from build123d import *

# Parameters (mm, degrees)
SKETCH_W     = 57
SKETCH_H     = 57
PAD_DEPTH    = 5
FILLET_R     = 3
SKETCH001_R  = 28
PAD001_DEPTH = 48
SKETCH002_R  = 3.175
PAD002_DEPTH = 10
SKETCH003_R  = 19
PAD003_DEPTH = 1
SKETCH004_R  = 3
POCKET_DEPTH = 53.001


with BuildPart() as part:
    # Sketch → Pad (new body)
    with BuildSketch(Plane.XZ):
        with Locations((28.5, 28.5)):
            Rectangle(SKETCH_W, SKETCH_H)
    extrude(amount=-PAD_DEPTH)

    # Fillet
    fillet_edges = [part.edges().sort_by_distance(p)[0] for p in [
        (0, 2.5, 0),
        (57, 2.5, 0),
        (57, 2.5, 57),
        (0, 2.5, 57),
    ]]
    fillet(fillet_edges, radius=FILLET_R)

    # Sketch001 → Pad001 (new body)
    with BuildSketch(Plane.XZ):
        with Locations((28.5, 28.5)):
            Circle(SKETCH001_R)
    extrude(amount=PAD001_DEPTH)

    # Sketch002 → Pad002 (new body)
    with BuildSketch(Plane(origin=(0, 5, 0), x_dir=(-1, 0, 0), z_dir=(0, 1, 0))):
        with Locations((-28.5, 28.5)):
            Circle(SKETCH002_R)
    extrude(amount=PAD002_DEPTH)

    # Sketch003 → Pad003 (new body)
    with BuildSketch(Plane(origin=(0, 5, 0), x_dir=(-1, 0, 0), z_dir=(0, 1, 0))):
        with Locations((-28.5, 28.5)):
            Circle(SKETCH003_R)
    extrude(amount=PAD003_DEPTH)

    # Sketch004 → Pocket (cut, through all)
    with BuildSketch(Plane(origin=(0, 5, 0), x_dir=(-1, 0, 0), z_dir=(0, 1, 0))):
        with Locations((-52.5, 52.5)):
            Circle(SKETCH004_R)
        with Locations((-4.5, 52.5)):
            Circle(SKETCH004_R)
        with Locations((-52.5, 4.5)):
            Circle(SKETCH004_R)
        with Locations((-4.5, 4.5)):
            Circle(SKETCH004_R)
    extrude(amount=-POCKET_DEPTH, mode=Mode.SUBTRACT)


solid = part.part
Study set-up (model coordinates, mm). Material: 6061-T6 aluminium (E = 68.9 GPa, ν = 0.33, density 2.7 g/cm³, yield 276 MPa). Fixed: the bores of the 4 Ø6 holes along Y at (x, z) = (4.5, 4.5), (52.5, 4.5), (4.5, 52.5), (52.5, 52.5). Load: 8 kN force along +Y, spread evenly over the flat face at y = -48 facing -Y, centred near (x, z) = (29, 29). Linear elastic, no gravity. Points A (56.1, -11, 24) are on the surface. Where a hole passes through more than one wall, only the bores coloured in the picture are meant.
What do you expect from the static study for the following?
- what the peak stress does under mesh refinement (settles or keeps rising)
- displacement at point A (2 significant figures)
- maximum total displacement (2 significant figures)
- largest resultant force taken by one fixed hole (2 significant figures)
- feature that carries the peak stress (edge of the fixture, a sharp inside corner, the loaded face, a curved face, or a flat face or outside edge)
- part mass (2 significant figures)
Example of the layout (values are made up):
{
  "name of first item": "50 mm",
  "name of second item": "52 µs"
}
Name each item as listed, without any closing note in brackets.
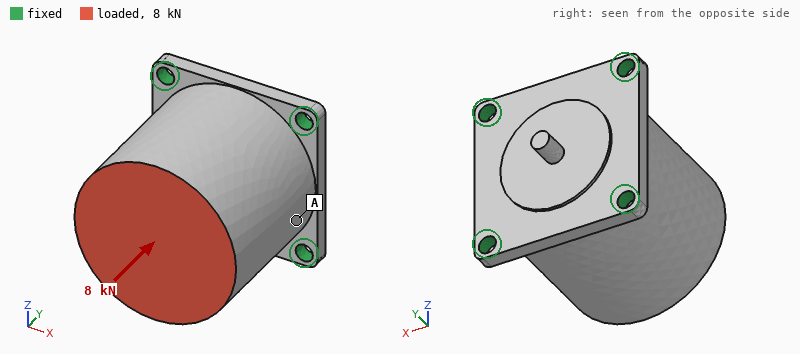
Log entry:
{
  "what the peak stress does under mesh refinement": "keeps rising",
  "displacement at point A": "14 µm",
  "maximum total displacement": "16 µm",
  "largest resultant force taken by one fixed hole": "2.2 kN",
  "feature that carries the peak stress": "edge of the fixture",
  "part mass": "370 g"
}
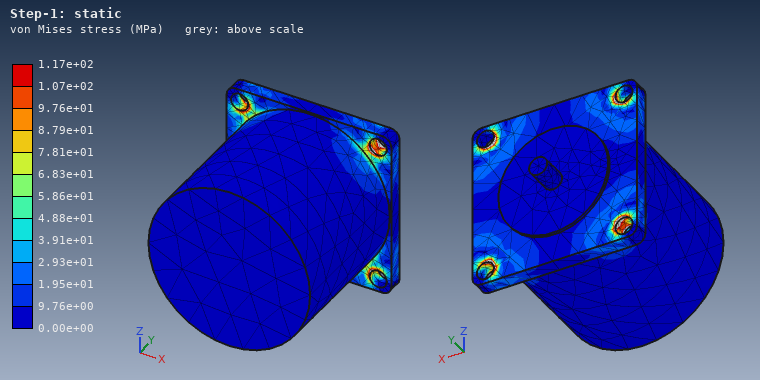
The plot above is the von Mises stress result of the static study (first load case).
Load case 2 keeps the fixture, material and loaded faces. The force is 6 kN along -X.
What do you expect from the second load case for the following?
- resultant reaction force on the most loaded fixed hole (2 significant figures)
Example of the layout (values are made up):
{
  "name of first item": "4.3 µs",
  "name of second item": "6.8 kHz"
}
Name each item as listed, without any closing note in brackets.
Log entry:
{
  "resultant reaction force on the most loaded fixed hole": "4.0 kN"
}
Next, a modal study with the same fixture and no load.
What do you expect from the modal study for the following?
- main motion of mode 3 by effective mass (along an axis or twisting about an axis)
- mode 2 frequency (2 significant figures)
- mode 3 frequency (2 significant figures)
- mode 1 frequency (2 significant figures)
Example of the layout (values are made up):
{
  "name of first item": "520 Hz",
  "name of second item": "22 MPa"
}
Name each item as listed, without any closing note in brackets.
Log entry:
{
  "main motion of mode 3 by effective mass": "along Y",
  "mode 2 frequency": "4000 Hz",
  "mode 3 frequency": "6200 Hz",
  "mode 1 frequency": "4000 Hz"
}
